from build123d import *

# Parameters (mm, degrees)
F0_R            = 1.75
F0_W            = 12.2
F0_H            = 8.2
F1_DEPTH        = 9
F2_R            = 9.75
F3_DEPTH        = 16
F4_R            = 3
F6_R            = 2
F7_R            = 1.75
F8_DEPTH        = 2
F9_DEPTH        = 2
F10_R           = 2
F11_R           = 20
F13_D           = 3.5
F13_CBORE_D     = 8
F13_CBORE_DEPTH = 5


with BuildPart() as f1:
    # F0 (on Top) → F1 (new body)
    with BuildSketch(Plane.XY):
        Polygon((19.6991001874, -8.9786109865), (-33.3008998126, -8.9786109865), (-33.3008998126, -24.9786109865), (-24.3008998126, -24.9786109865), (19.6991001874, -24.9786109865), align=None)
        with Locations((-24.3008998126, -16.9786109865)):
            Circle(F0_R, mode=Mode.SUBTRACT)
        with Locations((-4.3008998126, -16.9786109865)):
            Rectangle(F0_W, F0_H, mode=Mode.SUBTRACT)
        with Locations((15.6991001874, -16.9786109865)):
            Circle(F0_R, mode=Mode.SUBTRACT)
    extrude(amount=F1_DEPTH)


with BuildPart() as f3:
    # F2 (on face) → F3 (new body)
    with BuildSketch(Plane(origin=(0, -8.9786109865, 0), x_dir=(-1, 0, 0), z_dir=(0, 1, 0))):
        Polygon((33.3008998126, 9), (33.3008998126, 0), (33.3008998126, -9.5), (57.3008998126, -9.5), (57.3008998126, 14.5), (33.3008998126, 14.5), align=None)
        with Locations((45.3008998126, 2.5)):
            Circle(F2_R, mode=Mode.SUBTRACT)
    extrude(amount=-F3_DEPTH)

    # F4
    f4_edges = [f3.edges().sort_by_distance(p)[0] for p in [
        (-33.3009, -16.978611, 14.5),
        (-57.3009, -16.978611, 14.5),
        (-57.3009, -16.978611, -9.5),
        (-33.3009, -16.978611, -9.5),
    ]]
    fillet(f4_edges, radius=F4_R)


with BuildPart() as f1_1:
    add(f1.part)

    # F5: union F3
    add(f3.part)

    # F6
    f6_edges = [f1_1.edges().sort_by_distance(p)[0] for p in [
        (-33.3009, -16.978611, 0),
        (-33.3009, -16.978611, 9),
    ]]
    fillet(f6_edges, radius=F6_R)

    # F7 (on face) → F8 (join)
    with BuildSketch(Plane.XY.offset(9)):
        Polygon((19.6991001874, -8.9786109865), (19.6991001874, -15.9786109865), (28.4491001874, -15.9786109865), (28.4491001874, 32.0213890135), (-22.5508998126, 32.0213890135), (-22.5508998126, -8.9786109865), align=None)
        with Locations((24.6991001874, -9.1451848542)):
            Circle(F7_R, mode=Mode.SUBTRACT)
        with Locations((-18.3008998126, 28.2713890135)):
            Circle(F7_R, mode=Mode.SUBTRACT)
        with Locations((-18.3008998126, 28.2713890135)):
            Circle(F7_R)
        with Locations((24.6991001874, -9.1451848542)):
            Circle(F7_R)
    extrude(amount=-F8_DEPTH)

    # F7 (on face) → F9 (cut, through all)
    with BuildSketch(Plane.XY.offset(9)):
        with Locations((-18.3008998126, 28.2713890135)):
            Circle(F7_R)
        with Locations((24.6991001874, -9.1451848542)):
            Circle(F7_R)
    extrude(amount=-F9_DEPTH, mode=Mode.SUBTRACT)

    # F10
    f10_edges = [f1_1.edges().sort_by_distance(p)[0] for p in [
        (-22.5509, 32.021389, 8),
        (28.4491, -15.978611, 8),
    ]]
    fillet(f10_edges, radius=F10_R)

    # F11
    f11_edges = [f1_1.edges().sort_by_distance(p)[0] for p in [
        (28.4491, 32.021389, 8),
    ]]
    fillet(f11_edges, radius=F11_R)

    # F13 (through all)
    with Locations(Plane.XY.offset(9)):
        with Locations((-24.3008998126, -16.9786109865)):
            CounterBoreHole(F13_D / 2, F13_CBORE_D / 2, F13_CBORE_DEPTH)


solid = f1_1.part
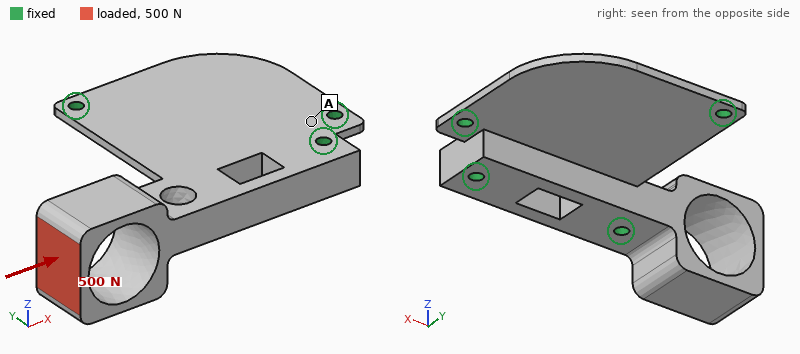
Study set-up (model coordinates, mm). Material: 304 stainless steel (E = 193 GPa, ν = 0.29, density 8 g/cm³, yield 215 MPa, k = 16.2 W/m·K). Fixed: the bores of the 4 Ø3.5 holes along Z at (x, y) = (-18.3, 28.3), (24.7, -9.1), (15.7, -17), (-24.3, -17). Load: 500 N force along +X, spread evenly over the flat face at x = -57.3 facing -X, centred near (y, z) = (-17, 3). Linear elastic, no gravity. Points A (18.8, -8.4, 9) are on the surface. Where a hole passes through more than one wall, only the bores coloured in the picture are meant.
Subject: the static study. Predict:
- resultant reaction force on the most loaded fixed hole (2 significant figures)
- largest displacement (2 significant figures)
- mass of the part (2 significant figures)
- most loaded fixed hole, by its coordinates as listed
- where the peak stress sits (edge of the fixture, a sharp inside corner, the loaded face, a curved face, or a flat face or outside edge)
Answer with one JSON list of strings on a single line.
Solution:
["440 N", "15 µm", "120 g", "(-24.3, -17)", "a curved face"]
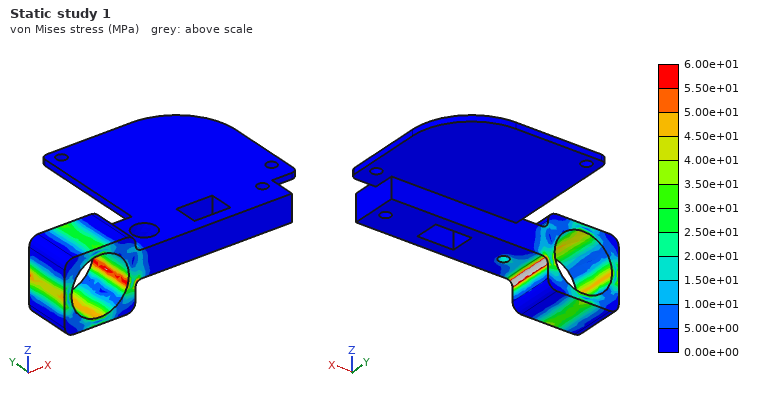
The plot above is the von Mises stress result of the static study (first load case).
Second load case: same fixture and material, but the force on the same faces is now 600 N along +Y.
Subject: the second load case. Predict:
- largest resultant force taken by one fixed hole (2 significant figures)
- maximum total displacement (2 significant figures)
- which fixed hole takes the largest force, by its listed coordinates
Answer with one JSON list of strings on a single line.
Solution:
["990 N", "50 µm", "(-24.3, -17)"]
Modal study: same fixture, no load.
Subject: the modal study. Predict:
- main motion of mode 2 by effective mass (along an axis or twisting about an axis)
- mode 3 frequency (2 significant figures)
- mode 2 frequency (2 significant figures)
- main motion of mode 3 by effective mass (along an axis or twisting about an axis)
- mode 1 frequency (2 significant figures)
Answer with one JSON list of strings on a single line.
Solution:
["along Z", "4800 Hz", "2900 Hz", "along Y", "2000 Hz"]
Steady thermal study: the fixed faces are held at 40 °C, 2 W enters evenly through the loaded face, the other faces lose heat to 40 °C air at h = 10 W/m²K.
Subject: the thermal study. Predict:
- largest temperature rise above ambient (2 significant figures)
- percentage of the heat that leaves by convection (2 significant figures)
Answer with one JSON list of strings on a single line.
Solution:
["36 K", "31 %"]
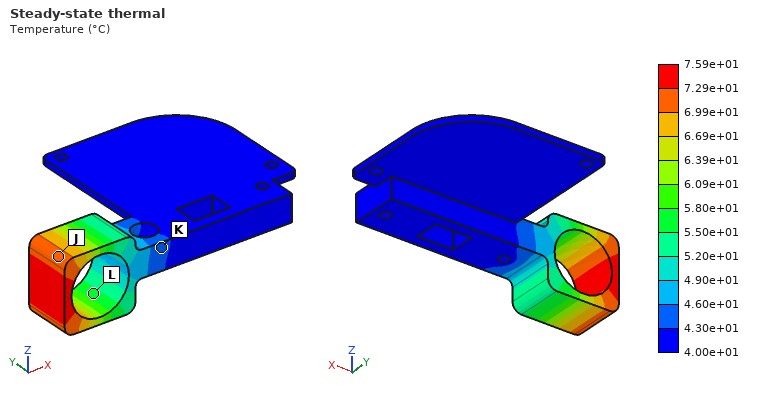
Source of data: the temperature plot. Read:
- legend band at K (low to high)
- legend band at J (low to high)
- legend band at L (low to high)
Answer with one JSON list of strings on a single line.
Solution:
["4.30e+01 to 4.60e+01 °C", "6.99e+01 to 7.29e+01 °C", "5.50e+01 to 5.80e+01 °C"]
